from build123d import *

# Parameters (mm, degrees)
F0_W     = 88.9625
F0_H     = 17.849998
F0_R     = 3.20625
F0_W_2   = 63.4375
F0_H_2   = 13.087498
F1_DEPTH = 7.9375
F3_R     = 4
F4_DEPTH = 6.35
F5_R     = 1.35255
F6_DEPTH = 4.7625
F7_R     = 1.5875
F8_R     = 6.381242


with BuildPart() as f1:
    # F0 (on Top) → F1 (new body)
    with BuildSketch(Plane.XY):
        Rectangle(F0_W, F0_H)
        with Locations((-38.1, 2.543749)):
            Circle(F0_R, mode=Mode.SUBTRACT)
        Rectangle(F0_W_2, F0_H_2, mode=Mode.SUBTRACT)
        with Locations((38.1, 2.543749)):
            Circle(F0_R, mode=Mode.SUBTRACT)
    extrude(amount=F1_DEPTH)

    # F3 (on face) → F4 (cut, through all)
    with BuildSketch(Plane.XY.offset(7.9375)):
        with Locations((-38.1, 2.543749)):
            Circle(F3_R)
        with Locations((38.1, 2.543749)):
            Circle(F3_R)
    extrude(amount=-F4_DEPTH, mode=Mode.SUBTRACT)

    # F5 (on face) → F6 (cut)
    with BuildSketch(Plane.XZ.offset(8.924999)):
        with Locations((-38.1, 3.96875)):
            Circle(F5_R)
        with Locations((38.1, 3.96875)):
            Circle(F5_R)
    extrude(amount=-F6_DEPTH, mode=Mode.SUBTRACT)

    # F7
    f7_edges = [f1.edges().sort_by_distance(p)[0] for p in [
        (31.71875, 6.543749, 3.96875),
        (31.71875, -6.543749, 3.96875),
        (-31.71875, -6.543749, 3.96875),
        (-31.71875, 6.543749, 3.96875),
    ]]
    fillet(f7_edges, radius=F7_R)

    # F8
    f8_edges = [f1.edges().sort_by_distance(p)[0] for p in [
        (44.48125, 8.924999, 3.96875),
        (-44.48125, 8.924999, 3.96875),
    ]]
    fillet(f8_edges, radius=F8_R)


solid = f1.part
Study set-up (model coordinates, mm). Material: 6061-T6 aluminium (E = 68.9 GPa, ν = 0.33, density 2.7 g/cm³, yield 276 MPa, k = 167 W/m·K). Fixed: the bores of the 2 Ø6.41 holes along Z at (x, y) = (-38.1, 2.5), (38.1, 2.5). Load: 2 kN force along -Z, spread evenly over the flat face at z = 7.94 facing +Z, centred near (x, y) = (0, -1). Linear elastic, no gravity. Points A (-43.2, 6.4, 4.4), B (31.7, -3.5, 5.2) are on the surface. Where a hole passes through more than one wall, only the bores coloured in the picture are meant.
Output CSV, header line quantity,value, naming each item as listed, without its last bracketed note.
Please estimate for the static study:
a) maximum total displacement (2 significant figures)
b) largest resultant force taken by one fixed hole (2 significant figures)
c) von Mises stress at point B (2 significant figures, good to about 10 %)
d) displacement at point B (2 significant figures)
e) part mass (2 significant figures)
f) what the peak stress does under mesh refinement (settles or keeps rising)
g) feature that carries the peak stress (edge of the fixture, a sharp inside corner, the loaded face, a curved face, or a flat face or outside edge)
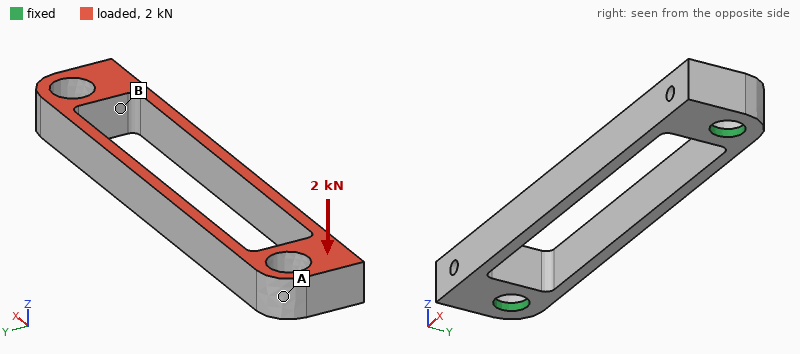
quantity,value
maximum total displacement,0.15 mm
largest resultant force taken by one fixed hole,1.1 kN
von Mises stress at point B,44 MPa
displacement at point B,0.028 mm
part mass,14 g
what the peak stress does under mesh refinement,keeps rising
feature that carries the peak stress,edge of the fixture
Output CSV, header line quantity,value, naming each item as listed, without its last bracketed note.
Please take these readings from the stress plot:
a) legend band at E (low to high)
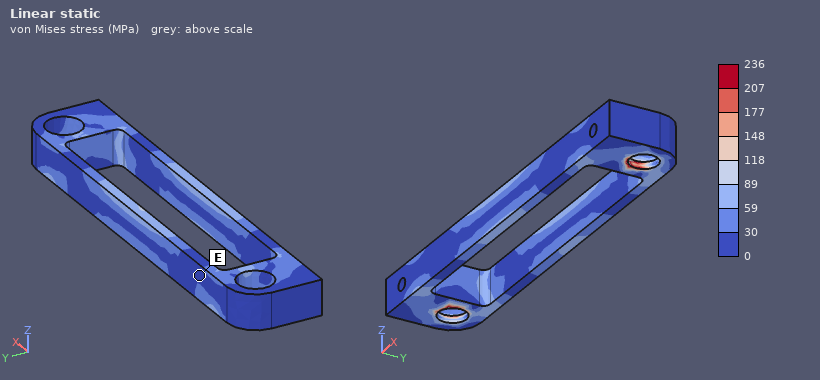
quantity,value
legend band at E,0 to 30 MPa
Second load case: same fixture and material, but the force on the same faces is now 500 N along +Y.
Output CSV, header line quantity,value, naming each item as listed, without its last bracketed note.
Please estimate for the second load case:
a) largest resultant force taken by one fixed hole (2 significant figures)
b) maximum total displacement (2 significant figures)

quantity,value
largest resultant force taken by one fixed hole,250 N
maximum total displacement,0.17 mm
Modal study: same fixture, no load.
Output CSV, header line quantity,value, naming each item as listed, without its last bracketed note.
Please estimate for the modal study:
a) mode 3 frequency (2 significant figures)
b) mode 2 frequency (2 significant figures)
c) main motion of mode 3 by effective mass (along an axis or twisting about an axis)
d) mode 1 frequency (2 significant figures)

quantity,value
mode 3 frequency,5900 Hz
mode 2 frequency,2900 Hz
main motion of mode 3 by effective mass,along Z
mode 1 frequency,2900 Hz
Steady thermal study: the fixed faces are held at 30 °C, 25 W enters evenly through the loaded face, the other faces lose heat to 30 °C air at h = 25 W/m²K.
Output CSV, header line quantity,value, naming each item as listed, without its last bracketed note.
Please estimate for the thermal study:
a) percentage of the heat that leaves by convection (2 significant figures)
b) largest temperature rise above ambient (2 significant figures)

quantity,value
percentage of the heat that leaves by convection,4.5 %
largest temperature rise above ambient,22 K
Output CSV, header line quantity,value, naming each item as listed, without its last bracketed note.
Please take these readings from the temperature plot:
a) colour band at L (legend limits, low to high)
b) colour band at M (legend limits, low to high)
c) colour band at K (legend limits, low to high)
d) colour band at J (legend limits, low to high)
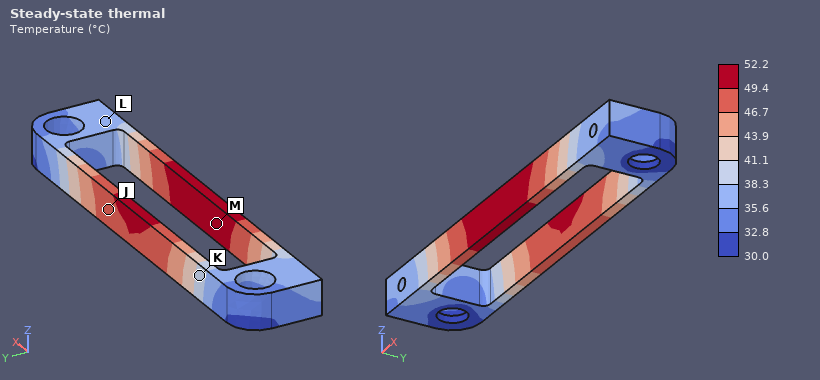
quantity,value
colour band at L,35.6 to 38.3 °C
colour band at M,49.4 to 52.2 °C
colour band at K,38.3 to 41.1 °C
colour band at J,46.7 to 49.4 °C
